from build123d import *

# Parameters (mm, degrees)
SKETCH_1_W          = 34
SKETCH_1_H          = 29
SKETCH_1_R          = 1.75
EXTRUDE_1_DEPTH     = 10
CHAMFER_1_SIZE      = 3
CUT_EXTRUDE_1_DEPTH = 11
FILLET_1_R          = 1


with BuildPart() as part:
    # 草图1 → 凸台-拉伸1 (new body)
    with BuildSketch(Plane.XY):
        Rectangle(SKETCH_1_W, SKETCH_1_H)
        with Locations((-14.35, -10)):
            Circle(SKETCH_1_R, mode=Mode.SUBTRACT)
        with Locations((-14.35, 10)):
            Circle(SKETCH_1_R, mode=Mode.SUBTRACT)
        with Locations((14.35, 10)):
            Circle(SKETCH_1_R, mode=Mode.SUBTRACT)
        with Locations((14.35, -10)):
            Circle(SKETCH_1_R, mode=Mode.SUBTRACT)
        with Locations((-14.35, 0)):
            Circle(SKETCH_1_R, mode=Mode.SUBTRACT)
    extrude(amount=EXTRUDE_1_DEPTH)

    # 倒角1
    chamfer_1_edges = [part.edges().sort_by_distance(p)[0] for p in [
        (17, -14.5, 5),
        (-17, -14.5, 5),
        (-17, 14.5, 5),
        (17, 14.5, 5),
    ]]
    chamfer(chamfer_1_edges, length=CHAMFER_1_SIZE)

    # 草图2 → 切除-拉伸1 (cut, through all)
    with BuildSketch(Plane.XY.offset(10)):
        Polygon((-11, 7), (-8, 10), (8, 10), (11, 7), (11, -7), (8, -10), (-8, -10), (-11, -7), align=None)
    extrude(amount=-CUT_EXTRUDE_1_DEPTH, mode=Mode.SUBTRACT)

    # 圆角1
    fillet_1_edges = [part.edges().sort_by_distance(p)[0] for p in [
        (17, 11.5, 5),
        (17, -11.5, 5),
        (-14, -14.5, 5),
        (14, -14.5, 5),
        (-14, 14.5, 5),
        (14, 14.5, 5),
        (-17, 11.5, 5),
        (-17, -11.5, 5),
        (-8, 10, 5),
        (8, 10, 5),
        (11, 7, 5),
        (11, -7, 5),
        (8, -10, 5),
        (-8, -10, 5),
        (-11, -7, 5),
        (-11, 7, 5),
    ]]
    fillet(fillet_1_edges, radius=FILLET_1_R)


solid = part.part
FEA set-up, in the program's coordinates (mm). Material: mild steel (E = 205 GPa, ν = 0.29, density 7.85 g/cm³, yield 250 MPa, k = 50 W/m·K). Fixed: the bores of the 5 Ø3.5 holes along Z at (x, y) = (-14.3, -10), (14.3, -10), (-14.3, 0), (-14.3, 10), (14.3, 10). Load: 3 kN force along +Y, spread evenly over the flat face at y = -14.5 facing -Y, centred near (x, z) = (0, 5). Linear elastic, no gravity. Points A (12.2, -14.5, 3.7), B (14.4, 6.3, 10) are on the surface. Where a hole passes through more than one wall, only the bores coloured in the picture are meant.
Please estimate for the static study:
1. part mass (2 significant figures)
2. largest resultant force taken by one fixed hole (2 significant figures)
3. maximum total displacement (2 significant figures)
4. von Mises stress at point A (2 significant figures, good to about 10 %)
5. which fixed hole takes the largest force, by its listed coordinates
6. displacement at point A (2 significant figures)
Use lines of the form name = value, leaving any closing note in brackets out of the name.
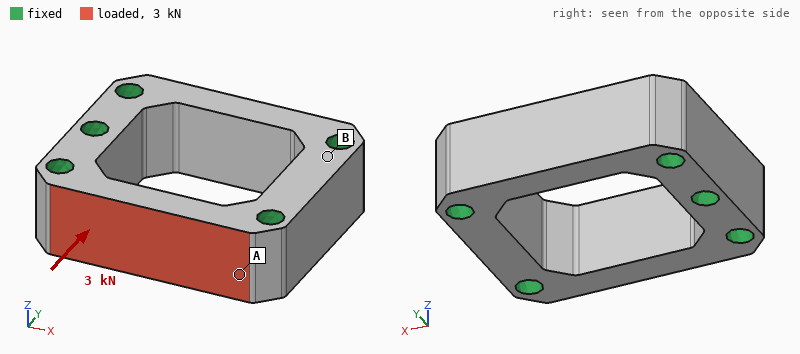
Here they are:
part mass = 39 g
largest resultant force taken by one fixed hole = 1.5 kN
maximum total displacement = 7.5 µm
von Mises stress at point A = 38 MPa
which fixed hole takes the largest force, by its listed coordinates = (14.3, -10)
displacement at point A = 1.5 µm
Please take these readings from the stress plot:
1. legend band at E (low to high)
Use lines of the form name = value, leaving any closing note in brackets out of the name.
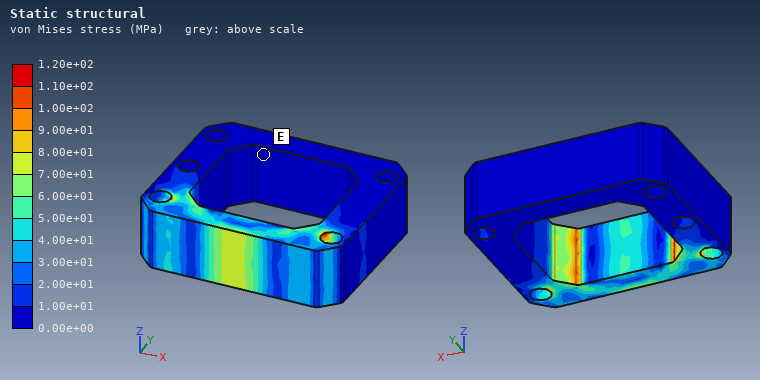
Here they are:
legend band at E = 0.00e+00 to 1.00e+01 MPa
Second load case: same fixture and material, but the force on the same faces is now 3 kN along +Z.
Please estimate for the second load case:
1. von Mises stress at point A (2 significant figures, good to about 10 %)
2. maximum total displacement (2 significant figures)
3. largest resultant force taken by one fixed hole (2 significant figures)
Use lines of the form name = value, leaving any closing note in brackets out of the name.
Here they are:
von Mises stress at point A = 64 MPa
maximum total displacement = 7.7 µm
largest resultant force taken by one fixed hole = 1.5 kN
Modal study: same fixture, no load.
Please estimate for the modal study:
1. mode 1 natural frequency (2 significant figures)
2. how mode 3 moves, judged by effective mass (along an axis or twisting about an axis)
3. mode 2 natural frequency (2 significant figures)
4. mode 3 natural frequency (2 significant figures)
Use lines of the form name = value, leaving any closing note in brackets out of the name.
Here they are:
mode 1 natural frequency = 37 kHz
how mode 3 moves, judged by effective mass = along Z
mode 2 natural frequency = 37 kHz
mode 3 natural frequency = 47 kHz
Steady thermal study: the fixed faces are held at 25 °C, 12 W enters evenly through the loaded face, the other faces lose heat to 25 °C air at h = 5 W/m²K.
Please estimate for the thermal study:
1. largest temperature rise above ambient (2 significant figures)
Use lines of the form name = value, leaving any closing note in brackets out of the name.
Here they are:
largest temperature rise above ambient = 17 K
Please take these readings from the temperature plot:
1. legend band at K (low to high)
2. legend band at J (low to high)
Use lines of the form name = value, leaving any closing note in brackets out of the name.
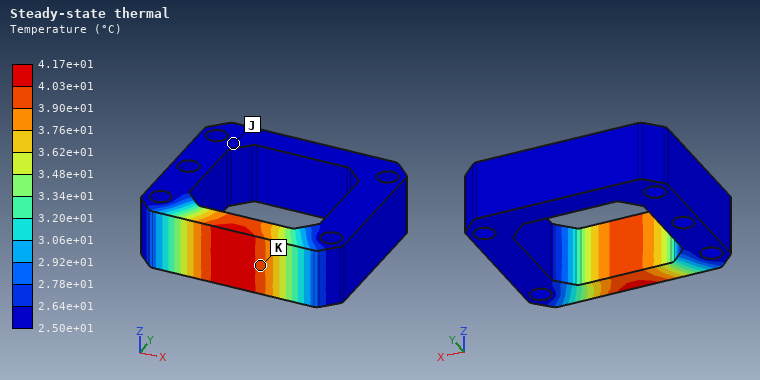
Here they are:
legend band at K = 3.90e+01 to 4.03e+01 °C
legend band at J = 2.50e+01 to 2.64e+01 °C
